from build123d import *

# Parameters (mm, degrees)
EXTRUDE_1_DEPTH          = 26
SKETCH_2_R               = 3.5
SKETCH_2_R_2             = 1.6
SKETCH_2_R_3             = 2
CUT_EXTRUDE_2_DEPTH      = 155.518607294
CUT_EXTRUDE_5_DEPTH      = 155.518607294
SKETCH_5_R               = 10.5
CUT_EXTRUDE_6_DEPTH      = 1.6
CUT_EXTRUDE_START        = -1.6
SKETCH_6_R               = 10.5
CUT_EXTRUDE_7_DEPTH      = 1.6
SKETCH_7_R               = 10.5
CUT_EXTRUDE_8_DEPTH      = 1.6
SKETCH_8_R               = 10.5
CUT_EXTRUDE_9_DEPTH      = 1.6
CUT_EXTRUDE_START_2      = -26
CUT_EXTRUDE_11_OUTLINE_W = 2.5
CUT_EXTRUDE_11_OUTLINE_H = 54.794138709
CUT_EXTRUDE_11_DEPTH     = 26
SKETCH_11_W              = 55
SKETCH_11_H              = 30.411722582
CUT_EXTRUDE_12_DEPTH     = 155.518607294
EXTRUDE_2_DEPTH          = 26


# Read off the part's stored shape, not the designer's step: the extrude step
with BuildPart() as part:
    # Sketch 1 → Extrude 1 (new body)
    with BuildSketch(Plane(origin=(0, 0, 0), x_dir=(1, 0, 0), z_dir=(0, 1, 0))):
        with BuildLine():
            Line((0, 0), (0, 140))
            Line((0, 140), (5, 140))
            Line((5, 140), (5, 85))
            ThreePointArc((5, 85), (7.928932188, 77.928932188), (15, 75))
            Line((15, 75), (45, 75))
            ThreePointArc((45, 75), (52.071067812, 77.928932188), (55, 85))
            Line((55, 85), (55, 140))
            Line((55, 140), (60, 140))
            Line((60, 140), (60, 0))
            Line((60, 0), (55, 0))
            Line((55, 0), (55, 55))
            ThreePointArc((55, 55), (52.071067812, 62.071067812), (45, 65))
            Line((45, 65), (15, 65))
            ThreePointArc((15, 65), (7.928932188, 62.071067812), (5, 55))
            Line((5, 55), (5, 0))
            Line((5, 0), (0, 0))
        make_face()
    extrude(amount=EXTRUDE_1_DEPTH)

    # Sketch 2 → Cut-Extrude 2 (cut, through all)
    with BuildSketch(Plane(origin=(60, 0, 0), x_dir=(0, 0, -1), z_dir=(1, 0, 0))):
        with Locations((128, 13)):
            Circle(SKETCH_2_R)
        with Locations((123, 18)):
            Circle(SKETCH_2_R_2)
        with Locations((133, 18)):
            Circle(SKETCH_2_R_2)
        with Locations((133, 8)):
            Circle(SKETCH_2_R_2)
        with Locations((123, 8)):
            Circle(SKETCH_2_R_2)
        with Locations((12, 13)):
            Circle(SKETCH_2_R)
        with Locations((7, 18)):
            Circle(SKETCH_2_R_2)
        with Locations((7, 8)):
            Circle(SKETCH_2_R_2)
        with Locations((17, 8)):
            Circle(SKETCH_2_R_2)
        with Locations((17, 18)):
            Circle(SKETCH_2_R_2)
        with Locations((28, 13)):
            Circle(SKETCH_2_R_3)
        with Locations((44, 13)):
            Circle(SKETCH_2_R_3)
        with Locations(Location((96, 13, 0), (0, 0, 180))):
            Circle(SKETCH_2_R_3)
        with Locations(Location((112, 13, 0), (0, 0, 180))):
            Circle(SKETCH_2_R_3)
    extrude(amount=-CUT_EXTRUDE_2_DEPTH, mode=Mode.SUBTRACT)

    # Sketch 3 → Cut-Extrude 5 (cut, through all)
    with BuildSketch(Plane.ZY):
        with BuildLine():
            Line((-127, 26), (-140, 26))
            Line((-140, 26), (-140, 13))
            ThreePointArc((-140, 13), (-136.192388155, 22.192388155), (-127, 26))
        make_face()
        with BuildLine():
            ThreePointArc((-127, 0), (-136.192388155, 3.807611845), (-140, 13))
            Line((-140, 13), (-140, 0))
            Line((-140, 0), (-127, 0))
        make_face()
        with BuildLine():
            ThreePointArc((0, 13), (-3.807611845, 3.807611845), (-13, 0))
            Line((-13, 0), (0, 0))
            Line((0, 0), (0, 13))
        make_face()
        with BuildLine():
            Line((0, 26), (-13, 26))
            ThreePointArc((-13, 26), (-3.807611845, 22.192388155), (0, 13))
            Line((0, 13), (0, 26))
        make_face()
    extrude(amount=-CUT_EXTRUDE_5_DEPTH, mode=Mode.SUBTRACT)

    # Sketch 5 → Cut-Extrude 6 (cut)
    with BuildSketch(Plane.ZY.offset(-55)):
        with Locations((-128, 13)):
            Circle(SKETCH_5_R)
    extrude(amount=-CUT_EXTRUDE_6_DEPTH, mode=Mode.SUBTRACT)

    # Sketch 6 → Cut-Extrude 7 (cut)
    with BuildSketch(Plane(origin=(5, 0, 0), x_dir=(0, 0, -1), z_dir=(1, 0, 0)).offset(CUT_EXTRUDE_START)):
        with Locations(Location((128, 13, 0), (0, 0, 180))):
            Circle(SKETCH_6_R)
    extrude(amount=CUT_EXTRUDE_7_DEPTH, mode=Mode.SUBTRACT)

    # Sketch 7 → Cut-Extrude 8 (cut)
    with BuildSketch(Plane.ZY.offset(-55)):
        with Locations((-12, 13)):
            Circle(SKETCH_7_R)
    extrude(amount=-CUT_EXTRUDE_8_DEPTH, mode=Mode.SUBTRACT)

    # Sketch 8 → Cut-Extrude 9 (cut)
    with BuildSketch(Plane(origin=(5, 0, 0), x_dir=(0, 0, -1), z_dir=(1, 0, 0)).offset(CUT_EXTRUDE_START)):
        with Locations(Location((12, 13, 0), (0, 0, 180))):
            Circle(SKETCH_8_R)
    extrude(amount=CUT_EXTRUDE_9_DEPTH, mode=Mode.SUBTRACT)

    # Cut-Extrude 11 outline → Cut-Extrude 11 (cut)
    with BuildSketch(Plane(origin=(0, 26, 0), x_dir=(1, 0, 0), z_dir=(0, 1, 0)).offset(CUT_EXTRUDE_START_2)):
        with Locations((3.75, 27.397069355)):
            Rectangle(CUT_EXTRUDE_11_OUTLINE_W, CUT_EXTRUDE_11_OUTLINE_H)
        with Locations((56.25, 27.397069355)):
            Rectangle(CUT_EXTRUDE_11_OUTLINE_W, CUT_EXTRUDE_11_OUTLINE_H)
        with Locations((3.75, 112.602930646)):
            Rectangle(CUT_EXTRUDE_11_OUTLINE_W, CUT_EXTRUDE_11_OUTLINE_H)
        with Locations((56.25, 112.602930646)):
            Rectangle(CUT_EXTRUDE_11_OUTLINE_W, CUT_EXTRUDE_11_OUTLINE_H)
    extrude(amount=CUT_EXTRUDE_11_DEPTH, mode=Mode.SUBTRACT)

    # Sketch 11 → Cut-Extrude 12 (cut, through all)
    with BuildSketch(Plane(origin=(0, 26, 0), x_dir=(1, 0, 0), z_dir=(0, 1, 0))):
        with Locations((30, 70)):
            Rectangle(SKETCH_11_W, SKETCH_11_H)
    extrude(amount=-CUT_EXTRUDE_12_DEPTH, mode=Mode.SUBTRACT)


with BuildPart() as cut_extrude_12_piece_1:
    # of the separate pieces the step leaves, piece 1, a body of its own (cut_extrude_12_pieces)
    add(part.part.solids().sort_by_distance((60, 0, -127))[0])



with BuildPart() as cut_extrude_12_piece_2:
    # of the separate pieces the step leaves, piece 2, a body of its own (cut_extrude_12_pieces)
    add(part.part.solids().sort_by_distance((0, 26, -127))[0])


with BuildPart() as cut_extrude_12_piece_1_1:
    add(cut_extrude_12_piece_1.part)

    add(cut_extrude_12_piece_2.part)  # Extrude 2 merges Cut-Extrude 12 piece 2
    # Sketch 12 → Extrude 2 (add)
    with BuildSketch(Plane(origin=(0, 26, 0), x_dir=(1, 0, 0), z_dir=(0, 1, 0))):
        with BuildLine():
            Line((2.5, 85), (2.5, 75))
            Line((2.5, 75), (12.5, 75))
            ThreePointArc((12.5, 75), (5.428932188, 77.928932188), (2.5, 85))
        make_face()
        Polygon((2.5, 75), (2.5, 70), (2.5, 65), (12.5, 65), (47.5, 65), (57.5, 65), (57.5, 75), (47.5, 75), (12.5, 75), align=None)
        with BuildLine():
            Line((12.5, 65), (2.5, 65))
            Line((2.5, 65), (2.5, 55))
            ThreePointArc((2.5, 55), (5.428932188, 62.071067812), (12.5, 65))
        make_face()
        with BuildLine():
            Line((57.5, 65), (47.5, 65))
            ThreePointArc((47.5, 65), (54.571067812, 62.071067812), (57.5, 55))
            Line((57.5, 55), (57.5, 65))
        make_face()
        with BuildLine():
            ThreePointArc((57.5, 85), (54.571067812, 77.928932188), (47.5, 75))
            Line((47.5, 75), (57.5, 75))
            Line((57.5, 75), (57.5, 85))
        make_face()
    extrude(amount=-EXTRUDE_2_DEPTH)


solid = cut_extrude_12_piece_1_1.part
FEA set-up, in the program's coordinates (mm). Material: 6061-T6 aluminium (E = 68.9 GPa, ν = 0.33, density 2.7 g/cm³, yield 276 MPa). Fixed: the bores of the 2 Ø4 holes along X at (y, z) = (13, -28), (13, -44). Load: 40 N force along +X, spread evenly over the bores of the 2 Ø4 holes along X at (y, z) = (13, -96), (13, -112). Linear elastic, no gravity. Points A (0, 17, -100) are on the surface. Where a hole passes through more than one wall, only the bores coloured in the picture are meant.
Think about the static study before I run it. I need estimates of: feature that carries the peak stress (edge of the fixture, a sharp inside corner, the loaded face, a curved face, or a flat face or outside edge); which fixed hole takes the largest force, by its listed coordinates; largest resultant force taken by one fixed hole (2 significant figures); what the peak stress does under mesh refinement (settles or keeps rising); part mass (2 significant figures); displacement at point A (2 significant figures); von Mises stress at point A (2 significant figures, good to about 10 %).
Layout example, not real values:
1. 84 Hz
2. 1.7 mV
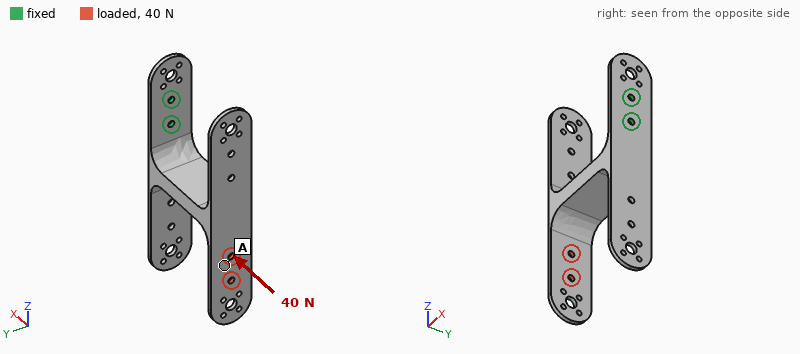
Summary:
1. edge of the fixture
2. (13, -44)
3. 86 N
4. keeps rising
5. 89 g
6. 1.1 mm
7. 8.9 MPa
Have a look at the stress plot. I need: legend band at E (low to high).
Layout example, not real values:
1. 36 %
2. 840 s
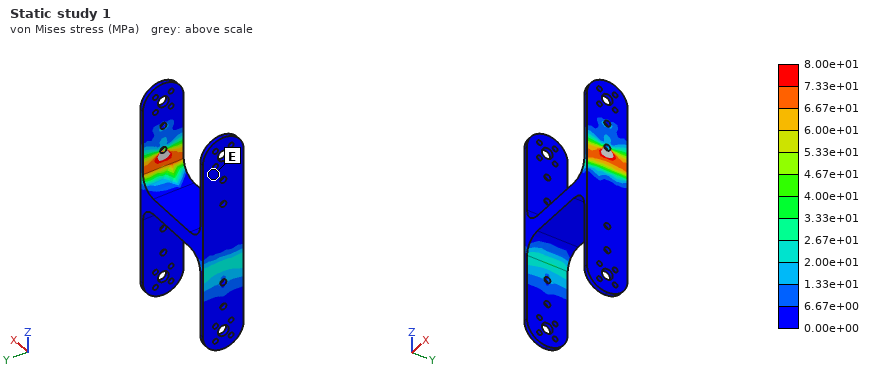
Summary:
1. 0.00e+00 to 6.67e+00 MPa
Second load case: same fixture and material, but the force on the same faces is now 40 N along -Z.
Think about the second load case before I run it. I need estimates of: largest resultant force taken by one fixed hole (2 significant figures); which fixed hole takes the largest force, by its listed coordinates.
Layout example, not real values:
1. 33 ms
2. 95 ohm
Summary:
1. 56 N
2. (13, -44)
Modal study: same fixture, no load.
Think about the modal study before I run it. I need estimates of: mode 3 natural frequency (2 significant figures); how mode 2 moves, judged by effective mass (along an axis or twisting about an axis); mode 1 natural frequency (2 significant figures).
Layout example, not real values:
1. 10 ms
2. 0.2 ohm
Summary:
1. 640 Hz
2. along Y
3. 140 Hz
